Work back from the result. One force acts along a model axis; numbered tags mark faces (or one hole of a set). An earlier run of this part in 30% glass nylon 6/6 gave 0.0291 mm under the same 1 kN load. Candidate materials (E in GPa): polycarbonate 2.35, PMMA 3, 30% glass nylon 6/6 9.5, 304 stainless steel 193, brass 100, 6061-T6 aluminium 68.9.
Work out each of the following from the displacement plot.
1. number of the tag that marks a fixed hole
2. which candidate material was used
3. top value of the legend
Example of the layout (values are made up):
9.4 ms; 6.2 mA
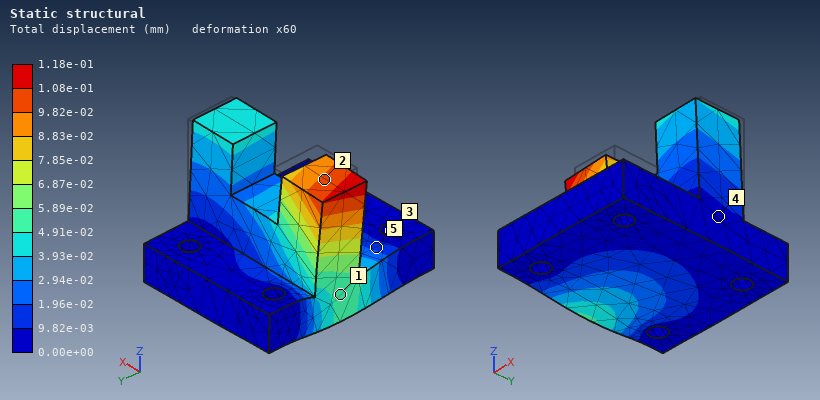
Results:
3; polycarbonate; 1.18e-01 mm
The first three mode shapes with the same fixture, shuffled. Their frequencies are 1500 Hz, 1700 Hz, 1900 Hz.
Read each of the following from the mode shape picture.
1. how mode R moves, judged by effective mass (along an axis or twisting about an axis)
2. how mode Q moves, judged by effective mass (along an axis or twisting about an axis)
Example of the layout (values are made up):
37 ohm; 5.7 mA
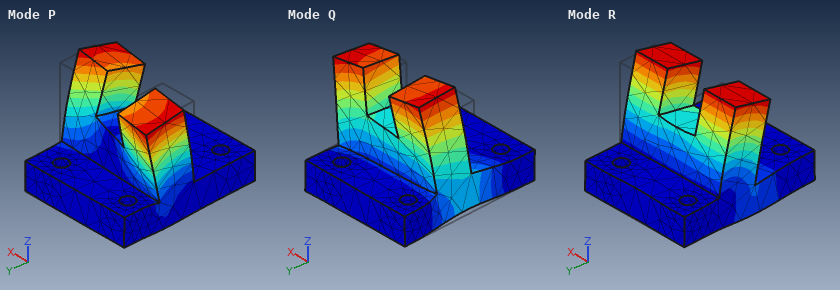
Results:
along Y; along X
